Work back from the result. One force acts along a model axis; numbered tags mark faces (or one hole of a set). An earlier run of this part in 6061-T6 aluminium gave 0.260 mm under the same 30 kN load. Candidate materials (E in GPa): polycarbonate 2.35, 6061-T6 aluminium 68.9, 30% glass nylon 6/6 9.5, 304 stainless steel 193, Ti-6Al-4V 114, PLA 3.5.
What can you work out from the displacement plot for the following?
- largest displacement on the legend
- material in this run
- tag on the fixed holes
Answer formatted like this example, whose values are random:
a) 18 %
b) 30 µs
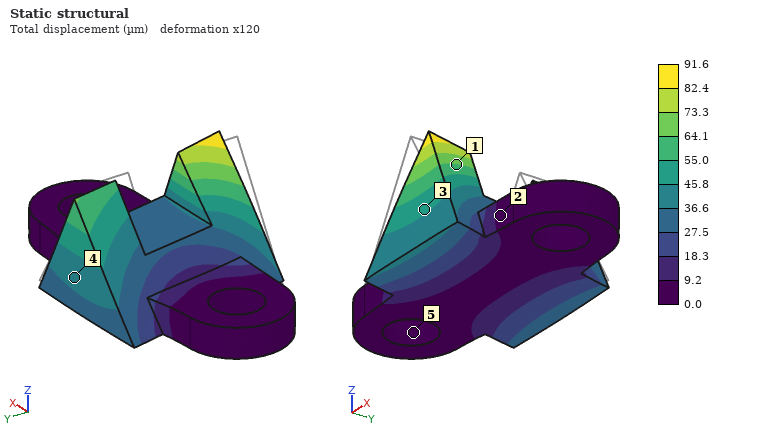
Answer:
a) 91.6 µm
b) 304 stainless steel
c) 5
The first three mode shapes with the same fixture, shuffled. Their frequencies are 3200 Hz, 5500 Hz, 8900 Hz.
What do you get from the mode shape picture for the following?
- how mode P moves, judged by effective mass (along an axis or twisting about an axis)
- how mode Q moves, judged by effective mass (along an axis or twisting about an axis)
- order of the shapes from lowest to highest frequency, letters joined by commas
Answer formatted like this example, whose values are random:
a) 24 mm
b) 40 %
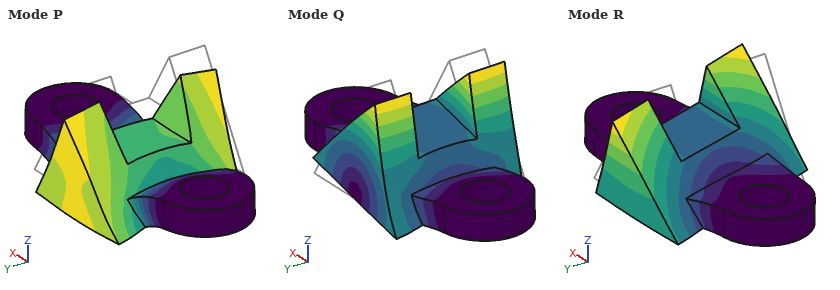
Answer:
a) along Z
b) along X
c) R, P, Q
